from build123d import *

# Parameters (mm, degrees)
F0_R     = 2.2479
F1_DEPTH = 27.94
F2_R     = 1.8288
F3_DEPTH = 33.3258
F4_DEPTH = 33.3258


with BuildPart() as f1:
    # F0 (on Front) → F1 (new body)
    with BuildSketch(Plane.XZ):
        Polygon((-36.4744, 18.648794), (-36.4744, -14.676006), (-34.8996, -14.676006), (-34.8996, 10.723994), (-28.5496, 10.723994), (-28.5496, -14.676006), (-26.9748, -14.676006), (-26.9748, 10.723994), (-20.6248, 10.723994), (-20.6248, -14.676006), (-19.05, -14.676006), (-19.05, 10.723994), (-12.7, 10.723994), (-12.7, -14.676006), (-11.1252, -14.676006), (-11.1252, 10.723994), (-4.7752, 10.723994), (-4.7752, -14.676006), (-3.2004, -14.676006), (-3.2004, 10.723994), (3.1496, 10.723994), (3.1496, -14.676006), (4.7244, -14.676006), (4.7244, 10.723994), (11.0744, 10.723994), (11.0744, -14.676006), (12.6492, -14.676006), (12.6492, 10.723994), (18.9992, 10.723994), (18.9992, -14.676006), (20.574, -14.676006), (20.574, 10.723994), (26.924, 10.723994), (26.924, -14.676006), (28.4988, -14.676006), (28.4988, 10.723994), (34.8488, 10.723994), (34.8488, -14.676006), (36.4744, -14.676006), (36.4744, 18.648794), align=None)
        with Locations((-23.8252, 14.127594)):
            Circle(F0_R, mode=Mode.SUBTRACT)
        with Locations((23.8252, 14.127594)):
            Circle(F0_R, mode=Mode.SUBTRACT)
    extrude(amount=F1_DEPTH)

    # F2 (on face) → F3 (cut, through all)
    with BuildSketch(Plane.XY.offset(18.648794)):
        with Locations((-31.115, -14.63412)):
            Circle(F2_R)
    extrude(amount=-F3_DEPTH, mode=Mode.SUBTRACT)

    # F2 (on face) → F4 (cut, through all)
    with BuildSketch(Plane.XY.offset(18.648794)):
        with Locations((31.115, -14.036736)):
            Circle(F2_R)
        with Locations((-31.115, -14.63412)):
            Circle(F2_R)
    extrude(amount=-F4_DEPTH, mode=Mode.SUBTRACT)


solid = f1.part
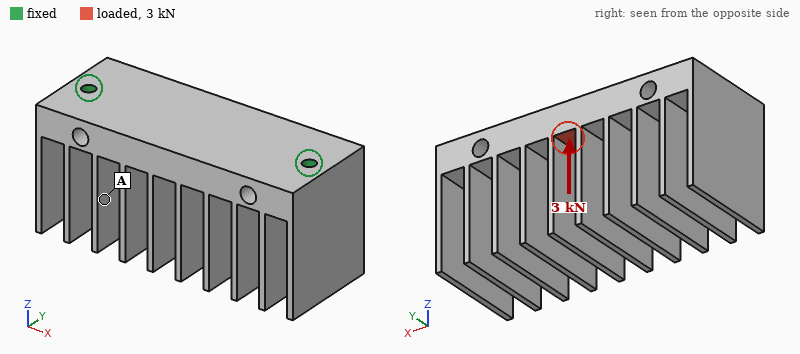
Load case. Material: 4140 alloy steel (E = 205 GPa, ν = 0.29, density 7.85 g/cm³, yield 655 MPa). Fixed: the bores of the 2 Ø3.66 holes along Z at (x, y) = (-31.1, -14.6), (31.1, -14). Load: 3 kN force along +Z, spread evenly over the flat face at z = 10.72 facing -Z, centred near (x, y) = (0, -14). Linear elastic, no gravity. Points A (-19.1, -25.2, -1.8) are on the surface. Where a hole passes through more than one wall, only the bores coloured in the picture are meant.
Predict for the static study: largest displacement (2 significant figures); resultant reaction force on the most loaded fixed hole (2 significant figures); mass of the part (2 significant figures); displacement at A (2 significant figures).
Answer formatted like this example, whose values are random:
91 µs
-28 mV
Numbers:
33 µm
1.5 kN
210 g
20 µm
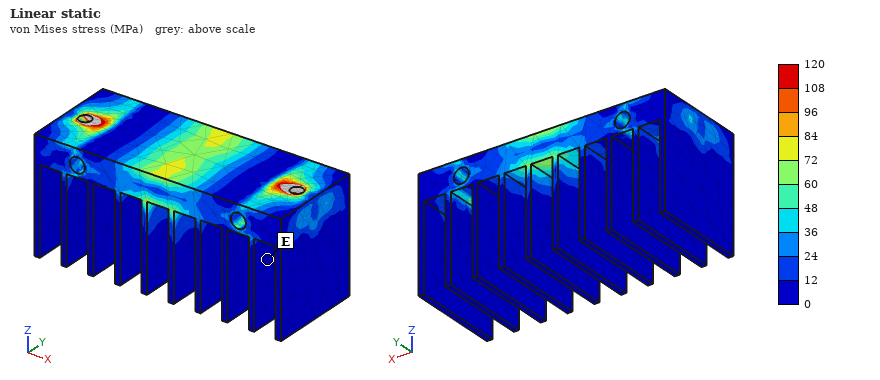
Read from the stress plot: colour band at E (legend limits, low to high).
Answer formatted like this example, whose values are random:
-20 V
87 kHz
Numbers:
0 to 12 MPa
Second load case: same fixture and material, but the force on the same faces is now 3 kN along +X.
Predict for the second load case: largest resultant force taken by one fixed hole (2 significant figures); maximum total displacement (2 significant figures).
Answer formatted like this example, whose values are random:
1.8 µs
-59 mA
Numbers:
1.5 kN
5.9 µm
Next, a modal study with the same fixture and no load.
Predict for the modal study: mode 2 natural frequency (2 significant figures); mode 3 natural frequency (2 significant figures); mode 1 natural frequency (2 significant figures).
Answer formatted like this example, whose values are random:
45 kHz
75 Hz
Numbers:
2000 Hz
2000 Hz
1900 Hz
